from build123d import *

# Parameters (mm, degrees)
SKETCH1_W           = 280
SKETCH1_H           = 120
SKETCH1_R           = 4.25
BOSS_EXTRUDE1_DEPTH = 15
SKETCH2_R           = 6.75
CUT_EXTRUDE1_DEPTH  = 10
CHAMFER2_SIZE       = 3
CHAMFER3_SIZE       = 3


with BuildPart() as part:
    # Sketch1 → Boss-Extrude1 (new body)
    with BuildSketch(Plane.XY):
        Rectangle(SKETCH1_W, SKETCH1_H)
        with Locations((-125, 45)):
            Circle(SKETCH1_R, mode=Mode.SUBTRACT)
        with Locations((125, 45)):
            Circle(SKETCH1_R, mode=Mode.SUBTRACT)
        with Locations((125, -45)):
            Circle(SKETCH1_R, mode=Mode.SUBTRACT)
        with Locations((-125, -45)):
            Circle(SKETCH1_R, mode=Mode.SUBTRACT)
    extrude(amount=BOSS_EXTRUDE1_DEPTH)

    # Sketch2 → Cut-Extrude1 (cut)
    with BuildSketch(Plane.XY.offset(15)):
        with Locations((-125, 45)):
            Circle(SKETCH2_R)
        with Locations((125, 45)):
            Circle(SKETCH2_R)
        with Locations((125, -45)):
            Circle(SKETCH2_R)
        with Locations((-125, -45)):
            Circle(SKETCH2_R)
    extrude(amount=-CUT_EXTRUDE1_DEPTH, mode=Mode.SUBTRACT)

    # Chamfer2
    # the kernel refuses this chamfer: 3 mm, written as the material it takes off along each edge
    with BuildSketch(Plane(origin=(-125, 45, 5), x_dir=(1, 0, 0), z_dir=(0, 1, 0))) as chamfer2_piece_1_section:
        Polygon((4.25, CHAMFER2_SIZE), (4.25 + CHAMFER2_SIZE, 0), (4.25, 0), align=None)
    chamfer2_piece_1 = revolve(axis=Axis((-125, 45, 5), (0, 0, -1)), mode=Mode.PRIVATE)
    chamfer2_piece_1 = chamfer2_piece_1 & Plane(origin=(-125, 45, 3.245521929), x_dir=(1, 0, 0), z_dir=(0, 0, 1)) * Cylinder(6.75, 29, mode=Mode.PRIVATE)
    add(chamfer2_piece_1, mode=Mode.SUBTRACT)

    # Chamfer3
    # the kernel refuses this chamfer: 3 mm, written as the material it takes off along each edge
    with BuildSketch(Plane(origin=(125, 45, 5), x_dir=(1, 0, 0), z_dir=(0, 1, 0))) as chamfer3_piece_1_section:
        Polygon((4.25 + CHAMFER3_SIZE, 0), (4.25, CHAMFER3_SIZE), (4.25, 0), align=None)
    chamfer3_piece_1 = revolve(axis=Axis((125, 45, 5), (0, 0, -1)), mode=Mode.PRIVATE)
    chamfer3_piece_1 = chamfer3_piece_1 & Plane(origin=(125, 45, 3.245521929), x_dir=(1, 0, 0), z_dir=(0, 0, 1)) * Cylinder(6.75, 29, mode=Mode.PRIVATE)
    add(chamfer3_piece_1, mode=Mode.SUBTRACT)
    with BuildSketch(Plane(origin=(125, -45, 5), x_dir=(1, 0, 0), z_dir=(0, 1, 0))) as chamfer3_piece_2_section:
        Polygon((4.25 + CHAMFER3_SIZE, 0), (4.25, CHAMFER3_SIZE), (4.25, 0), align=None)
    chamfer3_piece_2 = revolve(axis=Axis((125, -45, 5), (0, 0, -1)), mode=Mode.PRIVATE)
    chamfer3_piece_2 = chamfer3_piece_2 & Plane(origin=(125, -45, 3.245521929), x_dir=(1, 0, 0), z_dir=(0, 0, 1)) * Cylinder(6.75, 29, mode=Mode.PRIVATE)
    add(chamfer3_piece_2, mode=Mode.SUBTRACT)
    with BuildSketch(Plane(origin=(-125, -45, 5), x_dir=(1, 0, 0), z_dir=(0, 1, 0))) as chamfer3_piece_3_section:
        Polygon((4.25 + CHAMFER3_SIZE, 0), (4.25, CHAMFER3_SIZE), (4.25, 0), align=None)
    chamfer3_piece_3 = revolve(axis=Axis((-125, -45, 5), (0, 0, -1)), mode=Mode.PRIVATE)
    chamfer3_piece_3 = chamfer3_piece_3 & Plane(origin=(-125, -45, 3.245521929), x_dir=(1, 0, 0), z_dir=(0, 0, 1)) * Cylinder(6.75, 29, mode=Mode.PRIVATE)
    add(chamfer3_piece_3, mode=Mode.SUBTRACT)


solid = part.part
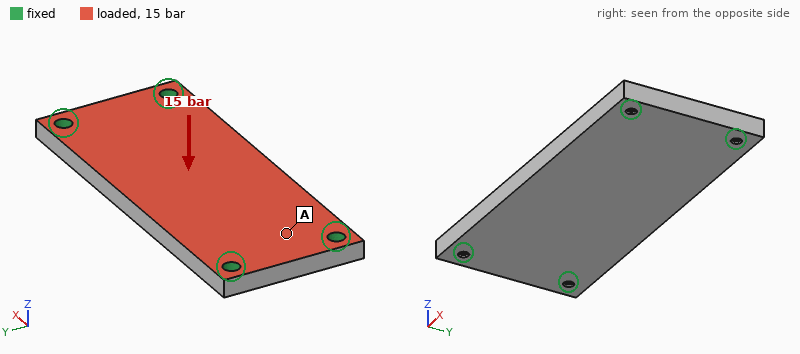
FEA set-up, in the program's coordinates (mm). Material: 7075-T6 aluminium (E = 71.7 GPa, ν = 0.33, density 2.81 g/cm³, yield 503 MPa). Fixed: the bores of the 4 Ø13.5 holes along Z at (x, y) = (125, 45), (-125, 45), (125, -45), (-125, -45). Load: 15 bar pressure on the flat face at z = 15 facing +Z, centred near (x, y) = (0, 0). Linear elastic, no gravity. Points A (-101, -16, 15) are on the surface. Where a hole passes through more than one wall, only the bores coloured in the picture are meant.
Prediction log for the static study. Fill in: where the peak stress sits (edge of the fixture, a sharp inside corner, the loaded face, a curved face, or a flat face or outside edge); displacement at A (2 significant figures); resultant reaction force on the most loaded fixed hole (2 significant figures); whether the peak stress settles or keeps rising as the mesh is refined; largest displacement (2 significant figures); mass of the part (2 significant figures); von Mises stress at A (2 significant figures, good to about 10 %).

edge of the fixture
0.19 mm
13 kN
keeps rising
0.97 mm
1.4 kg
66 MPa
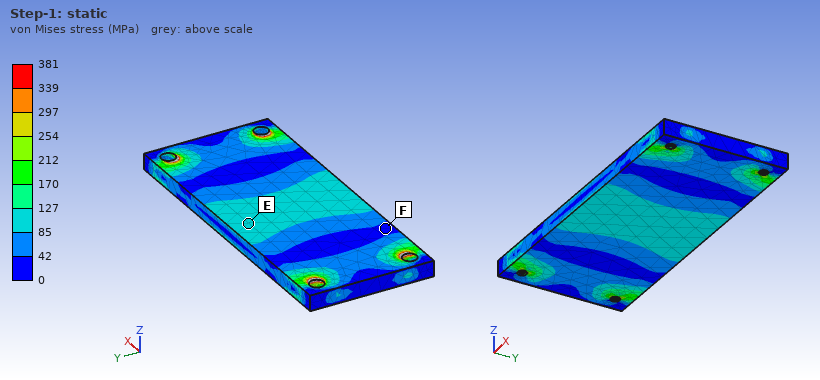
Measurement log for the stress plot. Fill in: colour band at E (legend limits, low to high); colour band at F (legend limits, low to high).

85 to 127 MPa
0 to 42 MPa
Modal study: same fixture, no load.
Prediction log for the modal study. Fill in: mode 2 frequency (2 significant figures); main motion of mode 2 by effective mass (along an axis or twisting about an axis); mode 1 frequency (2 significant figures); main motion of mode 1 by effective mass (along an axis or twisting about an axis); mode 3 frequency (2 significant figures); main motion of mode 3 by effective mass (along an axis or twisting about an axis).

2000 Hz
twisting about X
1100 Hz
along Z
3100 Hz
twisting about Y
